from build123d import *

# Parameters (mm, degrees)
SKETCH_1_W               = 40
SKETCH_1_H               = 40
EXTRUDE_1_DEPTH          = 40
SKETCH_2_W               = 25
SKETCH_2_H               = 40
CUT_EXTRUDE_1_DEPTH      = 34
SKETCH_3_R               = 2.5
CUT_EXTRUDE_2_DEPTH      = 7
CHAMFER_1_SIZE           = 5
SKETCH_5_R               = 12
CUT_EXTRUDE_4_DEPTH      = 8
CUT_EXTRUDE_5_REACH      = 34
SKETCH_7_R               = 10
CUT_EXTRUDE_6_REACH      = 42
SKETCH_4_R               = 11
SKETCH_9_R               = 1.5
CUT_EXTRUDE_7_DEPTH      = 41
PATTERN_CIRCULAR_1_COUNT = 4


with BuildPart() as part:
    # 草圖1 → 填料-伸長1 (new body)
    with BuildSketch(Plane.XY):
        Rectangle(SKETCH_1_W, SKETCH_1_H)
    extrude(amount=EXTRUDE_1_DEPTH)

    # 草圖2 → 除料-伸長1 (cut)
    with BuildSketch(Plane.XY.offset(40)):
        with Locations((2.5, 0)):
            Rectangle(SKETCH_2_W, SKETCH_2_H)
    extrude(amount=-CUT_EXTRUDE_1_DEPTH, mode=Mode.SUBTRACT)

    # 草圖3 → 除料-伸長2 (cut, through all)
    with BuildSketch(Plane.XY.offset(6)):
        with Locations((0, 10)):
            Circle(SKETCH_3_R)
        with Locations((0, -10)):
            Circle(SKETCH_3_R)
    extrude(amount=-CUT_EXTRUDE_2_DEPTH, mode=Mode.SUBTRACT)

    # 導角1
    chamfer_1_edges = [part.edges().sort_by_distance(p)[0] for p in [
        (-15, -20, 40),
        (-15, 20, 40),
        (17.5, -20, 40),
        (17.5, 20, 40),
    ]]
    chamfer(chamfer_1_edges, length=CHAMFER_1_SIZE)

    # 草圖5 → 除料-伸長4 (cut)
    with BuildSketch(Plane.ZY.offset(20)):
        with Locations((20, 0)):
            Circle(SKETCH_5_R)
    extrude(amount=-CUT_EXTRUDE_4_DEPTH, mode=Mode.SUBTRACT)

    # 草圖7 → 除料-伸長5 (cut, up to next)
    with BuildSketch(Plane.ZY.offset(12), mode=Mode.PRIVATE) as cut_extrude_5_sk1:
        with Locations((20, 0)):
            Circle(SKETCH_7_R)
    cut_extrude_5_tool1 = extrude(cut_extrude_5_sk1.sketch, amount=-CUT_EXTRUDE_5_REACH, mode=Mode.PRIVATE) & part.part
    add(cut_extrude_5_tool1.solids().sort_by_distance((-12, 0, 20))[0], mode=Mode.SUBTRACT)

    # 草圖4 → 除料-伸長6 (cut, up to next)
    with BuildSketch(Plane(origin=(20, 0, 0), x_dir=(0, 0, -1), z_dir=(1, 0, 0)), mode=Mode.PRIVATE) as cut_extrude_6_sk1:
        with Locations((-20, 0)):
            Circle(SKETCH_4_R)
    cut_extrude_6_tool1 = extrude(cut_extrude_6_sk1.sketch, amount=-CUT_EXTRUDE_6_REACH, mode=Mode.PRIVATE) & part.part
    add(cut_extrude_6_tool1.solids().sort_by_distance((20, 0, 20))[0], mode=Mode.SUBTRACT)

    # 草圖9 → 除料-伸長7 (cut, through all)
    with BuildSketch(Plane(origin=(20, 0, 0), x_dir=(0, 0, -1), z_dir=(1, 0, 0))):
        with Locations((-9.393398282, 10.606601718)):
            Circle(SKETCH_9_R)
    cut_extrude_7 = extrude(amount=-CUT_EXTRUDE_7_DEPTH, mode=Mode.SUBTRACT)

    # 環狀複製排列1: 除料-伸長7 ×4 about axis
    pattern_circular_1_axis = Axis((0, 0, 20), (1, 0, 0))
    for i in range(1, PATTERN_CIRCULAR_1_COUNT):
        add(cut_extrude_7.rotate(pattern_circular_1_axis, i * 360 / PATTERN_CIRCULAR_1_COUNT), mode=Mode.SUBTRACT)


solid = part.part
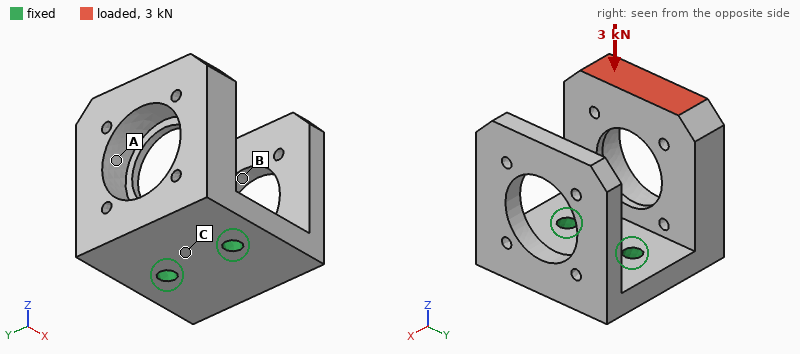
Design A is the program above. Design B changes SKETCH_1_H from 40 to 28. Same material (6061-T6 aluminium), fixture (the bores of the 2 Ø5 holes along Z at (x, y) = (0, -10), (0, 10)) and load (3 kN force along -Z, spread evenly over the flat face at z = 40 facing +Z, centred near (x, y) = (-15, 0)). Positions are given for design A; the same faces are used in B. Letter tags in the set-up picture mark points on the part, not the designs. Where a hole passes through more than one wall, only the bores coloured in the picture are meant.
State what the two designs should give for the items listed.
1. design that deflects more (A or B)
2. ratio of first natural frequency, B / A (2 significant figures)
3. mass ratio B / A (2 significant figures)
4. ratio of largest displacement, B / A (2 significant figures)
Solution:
B
0.91
0.61
1.4
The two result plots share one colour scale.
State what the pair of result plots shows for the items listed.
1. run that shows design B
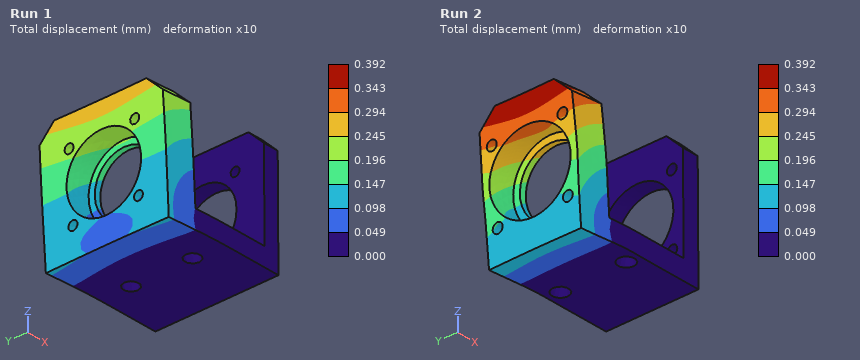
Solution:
Run 2
